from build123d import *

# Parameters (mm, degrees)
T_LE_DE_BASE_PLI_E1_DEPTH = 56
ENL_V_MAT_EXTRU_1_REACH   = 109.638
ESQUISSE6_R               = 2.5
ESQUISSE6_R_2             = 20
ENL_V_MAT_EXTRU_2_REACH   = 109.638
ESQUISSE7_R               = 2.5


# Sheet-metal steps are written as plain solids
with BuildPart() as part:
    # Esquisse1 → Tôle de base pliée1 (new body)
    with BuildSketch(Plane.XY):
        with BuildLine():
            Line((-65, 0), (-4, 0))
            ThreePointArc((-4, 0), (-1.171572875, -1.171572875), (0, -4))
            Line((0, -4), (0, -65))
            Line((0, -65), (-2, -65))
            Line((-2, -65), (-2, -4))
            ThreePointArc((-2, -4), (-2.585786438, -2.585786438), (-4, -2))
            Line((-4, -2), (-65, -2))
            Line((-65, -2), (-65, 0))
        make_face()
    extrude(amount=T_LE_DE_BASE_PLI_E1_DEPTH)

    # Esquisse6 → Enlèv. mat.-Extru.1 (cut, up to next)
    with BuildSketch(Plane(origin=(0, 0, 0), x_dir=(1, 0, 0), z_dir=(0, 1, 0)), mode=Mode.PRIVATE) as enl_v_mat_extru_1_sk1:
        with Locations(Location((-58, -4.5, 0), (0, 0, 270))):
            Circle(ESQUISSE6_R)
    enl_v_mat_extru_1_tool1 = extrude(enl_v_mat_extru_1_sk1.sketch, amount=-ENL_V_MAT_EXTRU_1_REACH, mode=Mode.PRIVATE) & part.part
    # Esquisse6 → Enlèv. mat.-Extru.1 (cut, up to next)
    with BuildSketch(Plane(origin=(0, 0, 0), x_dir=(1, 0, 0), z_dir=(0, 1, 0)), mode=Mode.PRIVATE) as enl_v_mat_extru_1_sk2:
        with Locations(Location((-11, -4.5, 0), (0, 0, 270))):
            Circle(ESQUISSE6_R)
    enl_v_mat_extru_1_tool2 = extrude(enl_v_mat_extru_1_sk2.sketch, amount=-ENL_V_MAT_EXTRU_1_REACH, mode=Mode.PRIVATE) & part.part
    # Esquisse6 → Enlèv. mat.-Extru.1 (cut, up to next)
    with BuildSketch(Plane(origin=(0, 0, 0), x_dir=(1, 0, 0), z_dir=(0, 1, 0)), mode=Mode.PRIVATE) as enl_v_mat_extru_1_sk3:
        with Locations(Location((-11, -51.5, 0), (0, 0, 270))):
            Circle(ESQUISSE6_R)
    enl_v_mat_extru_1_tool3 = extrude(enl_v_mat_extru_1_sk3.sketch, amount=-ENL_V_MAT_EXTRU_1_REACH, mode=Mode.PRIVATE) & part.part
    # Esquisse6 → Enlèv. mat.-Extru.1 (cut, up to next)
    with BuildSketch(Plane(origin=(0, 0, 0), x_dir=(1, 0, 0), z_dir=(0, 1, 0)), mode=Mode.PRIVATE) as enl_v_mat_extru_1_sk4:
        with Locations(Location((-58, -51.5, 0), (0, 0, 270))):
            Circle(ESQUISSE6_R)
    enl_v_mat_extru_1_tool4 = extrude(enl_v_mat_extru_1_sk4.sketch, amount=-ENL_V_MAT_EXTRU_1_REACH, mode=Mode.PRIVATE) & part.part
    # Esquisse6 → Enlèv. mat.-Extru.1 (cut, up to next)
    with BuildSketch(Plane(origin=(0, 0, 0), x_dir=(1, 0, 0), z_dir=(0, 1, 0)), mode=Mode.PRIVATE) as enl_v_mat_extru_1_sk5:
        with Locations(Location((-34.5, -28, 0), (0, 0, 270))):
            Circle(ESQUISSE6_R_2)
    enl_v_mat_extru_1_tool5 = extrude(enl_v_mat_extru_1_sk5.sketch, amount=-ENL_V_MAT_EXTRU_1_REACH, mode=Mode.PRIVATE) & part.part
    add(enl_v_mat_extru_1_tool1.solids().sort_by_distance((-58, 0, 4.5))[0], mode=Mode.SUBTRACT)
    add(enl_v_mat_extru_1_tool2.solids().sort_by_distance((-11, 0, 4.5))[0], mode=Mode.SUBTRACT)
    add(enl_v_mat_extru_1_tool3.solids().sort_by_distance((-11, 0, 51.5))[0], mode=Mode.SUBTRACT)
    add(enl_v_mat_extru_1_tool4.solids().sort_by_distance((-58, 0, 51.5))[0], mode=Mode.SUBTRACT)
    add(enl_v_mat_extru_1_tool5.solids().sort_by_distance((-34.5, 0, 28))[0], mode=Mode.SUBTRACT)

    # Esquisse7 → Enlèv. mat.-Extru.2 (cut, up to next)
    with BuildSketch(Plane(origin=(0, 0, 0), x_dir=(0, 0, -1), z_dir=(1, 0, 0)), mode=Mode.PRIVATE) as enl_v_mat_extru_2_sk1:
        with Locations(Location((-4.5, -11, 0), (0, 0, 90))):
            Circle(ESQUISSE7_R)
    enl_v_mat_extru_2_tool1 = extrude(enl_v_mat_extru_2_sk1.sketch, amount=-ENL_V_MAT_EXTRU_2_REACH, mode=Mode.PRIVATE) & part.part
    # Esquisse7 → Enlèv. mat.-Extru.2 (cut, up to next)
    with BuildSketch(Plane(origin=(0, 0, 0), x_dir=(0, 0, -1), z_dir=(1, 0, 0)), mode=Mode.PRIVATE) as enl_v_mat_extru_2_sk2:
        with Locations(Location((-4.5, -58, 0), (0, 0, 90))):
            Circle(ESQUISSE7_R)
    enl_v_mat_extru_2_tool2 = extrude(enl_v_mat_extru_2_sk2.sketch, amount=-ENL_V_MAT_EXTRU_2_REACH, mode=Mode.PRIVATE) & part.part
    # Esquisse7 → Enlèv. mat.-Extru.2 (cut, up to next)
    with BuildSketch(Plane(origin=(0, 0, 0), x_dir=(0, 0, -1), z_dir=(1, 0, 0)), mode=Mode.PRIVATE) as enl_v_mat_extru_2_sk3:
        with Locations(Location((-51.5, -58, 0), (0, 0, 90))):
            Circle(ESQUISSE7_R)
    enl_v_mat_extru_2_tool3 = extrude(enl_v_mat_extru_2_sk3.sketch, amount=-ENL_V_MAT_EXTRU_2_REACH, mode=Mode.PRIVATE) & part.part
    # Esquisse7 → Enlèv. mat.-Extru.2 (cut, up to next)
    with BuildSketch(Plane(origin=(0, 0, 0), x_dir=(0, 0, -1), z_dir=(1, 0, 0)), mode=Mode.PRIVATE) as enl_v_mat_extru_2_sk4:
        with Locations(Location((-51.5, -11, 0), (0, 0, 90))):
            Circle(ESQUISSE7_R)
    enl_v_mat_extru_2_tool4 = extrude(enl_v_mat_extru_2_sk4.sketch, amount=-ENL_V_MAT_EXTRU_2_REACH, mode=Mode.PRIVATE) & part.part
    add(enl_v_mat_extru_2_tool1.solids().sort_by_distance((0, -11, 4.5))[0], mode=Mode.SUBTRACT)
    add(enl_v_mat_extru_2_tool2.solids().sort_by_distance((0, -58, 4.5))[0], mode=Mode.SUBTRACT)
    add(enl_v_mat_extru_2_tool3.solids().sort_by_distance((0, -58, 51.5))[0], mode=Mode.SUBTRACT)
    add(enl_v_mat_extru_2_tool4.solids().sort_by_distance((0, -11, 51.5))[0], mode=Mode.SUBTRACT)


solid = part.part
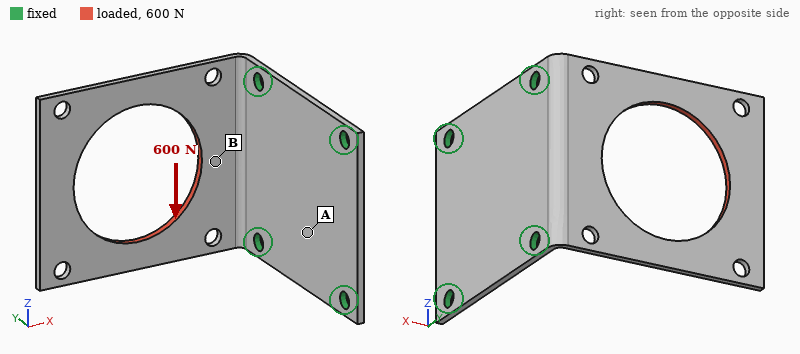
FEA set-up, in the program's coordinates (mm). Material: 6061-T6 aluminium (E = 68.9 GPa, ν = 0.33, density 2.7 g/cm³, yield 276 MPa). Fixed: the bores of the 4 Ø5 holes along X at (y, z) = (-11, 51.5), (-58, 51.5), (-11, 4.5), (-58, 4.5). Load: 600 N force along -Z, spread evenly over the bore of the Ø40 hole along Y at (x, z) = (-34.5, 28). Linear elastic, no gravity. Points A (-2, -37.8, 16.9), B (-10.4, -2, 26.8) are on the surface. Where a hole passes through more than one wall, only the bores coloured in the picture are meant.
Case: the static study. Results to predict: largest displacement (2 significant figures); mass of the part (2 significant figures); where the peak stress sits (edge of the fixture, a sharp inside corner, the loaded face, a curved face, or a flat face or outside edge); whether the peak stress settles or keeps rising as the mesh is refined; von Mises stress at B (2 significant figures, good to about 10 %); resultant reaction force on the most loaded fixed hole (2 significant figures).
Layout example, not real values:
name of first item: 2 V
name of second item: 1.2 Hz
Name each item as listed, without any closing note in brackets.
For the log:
largest displacement: 0.49 mm
mass of the part: 31 g
where the peak stress sits: edge of the fixture
whether the peak stress settles or keeps rising as the mesh is refined: keeps rising
von Mises stress at B: 67 MPa
resultant reaction force on the most loaded fixed hole: 540 N
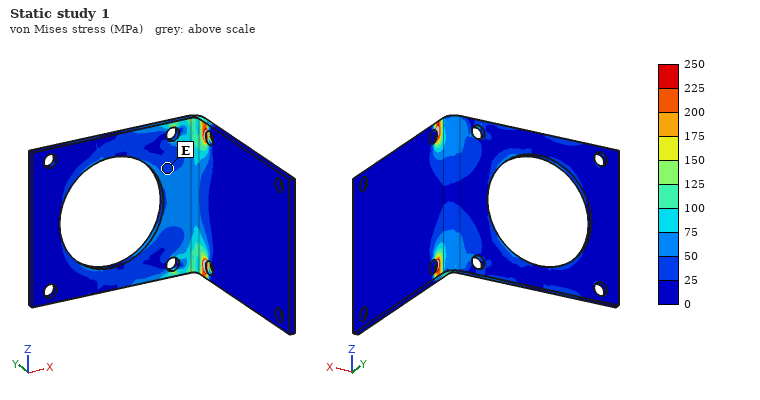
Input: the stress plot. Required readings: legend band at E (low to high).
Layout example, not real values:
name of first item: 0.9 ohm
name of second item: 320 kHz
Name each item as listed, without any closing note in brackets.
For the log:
legend band at E: 25 to 50 MPa
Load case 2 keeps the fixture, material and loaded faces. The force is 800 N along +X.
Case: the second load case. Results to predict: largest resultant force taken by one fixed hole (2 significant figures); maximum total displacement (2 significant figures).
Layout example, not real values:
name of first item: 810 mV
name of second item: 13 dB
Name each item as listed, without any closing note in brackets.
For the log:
largest resultant force taken by one fixed hole: 420 N
maximum total displacement: 0.94 mm
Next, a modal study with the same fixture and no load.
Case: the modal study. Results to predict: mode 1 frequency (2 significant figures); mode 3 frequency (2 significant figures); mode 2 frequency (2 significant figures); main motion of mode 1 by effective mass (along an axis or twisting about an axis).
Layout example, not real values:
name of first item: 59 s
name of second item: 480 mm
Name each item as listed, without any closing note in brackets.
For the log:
mode 1 frequency: 310 Hz
mode 3 frequency: 1900 Hz
mode 2 frequency: 820 Hz
main motion of mode 1 by effective mass: along Y
